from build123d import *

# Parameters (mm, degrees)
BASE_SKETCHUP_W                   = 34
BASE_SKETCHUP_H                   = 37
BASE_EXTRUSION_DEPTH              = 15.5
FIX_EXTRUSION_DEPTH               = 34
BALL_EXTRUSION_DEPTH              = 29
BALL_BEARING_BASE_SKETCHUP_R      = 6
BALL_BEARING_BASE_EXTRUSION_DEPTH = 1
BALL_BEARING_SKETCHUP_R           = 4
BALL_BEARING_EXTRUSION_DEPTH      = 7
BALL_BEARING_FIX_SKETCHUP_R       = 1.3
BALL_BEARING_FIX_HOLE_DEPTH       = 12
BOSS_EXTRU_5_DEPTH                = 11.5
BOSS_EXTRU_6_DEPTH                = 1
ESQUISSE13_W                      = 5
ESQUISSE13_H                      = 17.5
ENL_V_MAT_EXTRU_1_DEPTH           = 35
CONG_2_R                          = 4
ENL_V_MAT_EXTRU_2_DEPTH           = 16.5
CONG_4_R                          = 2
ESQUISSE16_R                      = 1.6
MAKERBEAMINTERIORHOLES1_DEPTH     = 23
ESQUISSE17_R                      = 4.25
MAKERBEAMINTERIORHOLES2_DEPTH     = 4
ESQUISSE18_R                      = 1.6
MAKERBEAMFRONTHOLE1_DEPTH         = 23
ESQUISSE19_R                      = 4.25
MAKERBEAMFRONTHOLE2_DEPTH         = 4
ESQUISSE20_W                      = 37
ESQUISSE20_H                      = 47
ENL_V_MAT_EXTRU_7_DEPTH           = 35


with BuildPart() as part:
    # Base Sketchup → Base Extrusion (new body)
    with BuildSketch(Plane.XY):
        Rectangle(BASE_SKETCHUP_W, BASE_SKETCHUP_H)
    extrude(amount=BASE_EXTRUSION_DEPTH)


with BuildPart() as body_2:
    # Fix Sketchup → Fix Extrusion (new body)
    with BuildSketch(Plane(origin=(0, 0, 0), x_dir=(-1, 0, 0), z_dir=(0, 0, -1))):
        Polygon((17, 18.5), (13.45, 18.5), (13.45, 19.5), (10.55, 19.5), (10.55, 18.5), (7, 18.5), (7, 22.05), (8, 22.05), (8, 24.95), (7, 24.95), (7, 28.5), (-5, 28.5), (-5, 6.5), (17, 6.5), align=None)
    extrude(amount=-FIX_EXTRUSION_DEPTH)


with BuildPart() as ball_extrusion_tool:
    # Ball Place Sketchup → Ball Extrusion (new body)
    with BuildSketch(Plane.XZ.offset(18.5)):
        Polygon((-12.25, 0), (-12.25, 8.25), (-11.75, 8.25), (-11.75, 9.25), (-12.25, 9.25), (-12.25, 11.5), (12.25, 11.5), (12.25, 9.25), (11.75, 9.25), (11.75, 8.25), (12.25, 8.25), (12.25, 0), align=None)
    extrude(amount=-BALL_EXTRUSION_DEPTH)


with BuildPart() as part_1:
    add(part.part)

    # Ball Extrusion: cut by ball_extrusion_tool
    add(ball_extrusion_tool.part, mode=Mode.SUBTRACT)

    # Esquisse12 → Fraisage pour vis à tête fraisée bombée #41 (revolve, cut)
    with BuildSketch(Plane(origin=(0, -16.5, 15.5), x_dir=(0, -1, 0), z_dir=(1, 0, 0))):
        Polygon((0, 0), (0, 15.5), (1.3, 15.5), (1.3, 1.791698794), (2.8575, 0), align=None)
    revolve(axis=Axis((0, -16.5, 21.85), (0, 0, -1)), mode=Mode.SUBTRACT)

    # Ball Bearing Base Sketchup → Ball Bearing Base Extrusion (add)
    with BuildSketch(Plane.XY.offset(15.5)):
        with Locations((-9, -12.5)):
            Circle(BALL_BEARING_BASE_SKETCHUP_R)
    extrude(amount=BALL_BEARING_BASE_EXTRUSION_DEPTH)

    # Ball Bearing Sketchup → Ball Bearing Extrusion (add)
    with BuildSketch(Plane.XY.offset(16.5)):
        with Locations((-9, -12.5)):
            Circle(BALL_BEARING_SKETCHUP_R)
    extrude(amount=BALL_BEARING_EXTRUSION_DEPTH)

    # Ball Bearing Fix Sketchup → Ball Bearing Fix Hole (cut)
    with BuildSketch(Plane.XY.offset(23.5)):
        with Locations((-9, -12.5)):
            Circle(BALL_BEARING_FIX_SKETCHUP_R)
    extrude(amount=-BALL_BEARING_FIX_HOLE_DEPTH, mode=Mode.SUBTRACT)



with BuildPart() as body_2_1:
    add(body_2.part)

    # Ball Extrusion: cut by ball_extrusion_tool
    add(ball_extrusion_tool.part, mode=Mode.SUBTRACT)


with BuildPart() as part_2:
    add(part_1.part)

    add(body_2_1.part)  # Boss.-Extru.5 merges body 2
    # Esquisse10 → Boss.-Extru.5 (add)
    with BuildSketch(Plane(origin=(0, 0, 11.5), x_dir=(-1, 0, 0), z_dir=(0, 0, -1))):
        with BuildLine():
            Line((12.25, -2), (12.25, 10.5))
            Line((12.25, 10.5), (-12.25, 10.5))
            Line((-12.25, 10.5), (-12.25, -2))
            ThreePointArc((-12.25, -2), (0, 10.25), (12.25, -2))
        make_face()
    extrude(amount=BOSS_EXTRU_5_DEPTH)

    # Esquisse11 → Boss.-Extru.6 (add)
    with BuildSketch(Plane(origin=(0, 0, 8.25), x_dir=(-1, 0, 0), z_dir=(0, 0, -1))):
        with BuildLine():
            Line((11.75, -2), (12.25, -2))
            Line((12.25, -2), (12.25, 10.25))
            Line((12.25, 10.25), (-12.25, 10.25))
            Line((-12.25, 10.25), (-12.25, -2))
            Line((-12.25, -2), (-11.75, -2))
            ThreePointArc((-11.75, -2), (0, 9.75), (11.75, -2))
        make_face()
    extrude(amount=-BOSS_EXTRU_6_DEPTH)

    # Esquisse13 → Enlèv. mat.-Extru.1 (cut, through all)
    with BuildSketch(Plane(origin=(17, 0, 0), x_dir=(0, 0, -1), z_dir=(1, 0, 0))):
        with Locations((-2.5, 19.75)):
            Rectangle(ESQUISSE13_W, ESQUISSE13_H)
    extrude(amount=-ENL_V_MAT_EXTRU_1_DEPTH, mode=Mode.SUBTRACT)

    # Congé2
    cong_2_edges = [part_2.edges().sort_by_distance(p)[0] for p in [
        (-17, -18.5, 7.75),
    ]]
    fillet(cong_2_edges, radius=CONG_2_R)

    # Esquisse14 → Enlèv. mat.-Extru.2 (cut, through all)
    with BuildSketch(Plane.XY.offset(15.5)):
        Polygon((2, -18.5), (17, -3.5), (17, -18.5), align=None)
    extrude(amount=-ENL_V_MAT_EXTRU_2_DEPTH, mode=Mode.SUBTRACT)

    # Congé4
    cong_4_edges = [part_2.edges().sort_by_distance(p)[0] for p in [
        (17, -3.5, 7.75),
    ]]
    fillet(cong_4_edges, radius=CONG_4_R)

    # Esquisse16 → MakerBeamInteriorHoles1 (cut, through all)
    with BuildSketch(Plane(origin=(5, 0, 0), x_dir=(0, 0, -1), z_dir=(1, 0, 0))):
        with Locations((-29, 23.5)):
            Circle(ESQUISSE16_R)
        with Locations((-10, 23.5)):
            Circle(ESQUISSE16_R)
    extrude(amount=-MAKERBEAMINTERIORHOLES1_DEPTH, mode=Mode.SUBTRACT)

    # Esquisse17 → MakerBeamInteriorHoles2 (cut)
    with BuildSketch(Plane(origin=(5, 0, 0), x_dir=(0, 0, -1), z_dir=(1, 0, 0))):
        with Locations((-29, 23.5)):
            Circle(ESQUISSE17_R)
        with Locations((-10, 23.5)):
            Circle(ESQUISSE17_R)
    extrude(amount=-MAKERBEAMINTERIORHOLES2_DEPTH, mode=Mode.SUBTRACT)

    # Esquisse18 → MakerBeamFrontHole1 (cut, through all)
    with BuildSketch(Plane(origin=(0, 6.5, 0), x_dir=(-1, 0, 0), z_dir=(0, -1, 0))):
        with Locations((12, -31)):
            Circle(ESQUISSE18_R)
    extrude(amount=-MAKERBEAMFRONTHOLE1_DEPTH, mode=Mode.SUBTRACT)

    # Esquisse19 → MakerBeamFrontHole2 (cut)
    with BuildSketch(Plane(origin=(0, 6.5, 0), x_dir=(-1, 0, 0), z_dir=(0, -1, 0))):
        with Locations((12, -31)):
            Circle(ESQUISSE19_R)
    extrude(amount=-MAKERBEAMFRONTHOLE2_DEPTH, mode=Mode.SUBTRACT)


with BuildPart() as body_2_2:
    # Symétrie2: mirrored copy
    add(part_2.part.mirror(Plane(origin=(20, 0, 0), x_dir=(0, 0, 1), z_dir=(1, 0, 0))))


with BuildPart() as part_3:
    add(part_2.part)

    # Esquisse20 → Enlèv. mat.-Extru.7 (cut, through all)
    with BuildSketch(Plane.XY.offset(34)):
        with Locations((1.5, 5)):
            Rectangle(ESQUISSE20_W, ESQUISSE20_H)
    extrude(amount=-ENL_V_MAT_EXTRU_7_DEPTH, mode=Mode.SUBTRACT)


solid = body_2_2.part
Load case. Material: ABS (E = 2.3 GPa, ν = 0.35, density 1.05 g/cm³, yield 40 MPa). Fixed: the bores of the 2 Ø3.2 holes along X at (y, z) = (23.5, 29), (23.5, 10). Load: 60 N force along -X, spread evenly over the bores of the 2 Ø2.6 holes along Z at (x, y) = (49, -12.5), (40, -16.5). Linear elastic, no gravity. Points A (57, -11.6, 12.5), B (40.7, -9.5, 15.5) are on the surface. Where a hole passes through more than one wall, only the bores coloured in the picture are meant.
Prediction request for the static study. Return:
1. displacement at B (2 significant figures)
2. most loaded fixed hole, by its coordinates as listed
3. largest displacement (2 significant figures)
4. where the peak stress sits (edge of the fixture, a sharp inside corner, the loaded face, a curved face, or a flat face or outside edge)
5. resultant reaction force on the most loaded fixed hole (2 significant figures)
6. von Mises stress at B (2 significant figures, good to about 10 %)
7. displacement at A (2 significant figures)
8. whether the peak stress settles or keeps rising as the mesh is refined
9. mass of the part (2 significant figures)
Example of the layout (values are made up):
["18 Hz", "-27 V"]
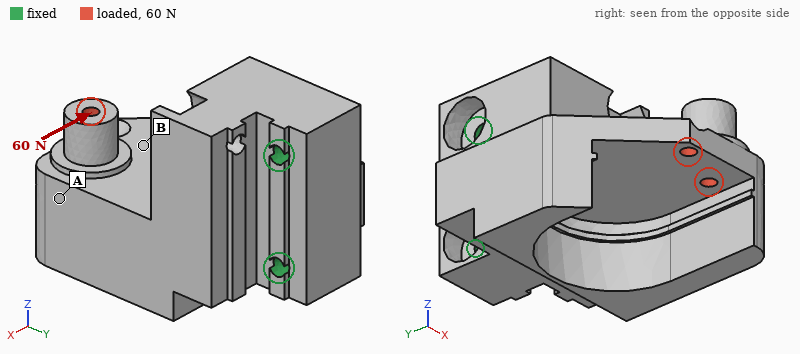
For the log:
["0.18 mm", "(23.5, 10)", "0.26 mm", "edge of the fixture", "36 N", "2.2 MPa", "0.21 mm", "keeps rising", "19 g"]
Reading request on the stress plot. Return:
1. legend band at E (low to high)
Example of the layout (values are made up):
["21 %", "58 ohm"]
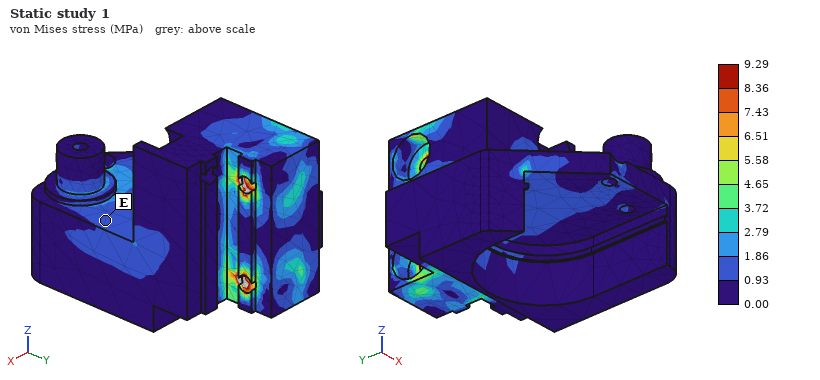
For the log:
["0.93 to 1.86 MPa"]
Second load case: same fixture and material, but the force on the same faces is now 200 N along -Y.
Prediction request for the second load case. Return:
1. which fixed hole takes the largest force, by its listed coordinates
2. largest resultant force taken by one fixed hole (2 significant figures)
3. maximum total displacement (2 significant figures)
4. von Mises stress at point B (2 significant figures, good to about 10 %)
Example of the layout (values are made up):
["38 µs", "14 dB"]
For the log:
["(23.5, 10)", "130 N", "0.24 mm", "3.6 MPa"]
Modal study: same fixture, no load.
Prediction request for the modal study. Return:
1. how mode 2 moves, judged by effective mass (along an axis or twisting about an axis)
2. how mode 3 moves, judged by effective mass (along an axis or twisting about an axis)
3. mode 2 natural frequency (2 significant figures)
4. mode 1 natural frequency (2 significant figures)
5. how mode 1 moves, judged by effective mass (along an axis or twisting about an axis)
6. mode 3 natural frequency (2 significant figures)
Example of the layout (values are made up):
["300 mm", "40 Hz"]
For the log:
["along Z", "twisting about Y", "2000 Hz", "1200 Hz", "along X", "3000 Hz"]
